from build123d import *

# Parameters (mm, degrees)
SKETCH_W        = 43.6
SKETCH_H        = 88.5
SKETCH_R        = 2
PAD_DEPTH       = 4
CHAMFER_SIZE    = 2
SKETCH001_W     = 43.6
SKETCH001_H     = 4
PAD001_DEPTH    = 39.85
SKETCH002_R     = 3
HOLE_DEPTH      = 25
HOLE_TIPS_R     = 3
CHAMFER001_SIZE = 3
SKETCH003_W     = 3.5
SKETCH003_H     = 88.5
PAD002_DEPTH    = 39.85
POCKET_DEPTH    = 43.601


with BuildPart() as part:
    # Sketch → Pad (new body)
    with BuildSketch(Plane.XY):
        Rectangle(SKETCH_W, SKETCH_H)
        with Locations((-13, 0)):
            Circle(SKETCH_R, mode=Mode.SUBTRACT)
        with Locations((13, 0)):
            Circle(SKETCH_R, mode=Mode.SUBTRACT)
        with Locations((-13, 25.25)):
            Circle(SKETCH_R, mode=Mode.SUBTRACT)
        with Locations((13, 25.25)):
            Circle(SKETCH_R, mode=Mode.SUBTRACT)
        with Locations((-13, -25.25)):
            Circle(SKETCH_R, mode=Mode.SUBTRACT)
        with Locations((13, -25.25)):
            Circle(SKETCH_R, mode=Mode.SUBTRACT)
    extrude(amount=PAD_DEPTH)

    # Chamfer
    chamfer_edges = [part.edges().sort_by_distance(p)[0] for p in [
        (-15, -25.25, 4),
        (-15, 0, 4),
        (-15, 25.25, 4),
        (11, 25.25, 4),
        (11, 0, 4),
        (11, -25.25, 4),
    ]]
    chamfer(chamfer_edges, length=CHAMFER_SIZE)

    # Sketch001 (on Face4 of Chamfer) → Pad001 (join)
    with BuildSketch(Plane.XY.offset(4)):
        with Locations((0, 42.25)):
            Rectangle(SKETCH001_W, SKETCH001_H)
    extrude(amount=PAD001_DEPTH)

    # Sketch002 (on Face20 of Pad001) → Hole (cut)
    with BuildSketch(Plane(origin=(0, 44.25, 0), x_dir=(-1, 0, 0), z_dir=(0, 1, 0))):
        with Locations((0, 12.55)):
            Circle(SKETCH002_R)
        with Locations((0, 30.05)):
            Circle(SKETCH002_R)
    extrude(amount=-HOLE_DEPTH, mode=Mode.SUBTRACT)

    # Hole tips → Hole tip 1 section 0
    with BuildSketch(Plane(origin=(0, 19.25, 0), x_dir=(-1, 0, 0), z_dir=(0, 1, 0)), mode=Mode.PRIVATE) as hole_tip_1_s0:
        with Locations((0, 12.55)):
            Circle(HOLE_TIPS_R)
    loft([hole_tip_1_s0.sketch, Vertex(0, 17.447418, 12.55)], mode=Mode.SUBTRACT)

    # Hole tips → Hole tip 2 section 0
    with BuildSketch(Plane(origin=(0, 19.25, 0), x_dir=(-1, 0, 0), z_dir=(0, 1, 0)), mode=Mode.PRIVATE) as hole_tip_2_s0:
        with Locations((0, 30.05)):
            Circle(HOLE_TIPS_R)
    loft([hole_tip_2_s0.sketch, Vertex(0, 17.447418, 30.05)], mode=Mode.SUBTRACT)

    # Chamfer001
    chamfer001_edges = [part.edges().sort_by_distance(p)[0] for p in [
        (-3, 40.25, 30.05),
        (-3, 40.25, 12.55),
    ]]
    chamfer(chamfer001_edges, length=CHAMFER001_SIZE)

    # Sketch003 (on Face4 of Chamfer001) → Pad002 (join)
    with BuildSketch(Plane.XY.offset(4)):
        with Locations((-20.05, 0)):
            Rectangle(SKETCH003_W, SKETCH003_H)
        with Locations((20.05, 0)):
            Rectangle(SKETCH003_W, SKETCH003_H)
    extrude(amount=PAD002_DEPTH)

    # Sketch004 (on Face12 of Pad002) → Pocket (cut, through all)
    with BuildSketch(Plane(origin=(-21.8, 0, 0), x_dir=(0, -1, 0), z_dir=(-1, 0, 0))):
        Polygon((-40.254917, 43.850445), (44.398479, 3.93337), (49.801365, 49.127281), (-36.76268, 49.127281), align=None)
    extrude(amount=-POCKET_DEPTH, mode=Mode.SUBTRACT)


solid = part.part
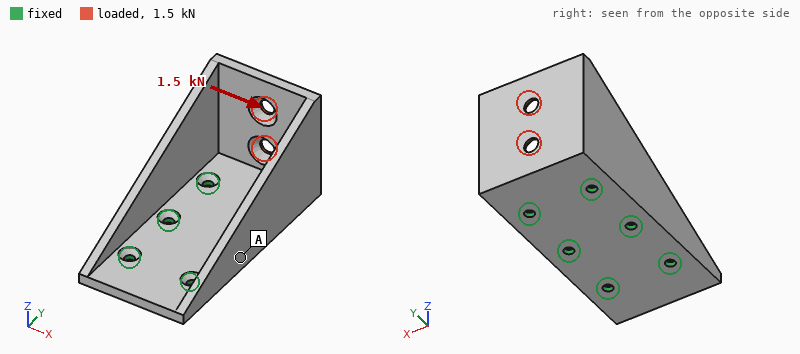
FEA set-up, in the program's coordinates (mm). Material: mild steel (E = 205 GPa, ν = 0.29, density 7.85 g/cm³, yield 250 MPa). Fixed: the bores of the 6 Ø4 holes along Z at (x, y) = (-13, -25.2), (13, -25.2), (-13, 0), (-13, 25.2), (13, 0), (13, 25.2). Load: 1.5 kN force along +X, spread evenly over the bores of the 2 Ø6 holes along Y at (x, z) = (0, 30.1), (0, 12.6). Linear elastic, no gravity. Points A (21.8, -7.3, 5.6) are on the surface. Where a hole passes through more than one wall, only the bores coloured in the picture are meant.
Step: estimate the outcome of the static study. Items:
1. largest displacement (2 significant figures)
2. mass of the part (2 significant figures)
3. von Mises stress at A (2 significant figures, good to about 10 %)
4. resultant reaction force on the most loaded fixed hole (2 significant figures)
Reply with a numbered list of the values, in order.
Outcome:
1. 39 µm
2. 260 g
3. 9.4 MPa
4. 1.6 kN
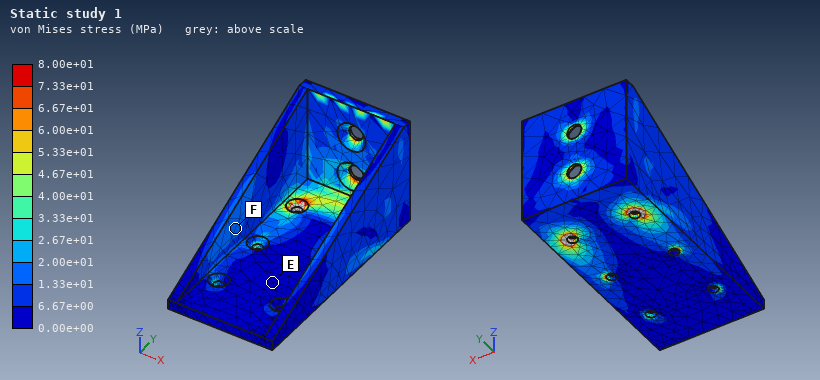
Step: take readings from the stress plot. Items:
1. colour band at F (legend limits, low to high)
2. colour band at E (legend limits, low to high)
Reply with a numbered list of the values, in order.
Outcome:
1. 1.33e+01 to 2.00e+01 MPa
2. 0.00e+00 to 6.67e+00 MPa
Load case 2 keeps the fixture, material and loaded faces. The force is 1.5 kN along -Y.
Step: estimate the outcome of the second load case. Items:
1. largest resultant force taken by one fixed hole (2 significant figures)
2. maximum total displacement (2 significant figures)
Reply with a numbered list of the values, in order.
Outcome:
1. 520 N
2. 35 µm
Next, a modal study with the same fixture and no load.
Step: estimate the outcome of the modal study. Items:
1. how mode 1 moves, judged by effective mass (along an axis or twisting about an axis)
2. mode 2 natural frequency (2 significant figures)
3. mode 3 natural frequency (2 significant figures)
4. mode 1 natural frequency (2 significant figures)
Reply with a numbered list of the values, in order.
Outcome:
1. along X
2. 4700 Hz
3. 5400 Hz
4. 3200 Hz
